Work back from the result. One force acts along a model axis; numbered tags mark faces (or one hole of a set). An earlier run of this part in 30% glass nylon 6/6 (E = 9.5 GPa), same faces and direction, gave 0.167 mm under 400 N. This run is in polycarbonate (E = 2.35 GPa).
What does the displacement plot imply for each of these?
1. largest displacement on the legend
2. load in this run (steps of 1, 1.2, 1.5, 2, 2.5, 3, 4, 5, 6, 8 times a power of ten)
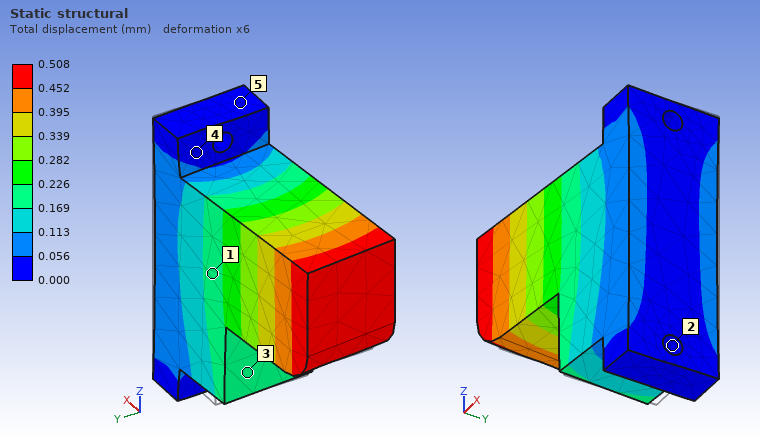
0.508 mm
300 N
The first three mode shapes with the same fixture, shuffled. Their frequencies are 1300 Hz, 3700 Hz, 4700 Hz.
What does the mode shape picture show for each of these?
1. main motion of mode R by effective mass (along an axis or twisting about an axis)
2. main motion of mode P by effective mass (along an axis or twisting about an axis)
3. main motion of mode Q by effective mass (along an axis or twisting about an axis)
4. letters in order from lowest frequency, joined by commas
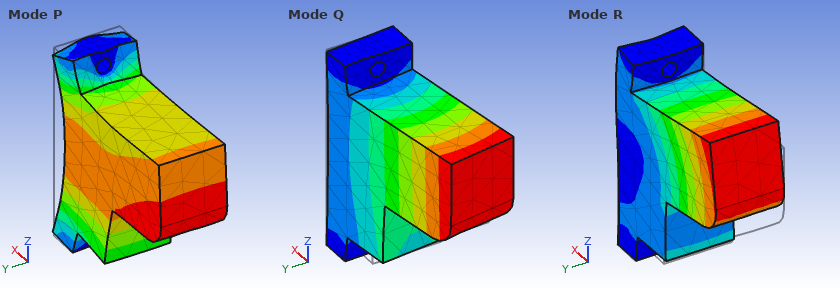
along Z
along X
along Y
Q, R, P
